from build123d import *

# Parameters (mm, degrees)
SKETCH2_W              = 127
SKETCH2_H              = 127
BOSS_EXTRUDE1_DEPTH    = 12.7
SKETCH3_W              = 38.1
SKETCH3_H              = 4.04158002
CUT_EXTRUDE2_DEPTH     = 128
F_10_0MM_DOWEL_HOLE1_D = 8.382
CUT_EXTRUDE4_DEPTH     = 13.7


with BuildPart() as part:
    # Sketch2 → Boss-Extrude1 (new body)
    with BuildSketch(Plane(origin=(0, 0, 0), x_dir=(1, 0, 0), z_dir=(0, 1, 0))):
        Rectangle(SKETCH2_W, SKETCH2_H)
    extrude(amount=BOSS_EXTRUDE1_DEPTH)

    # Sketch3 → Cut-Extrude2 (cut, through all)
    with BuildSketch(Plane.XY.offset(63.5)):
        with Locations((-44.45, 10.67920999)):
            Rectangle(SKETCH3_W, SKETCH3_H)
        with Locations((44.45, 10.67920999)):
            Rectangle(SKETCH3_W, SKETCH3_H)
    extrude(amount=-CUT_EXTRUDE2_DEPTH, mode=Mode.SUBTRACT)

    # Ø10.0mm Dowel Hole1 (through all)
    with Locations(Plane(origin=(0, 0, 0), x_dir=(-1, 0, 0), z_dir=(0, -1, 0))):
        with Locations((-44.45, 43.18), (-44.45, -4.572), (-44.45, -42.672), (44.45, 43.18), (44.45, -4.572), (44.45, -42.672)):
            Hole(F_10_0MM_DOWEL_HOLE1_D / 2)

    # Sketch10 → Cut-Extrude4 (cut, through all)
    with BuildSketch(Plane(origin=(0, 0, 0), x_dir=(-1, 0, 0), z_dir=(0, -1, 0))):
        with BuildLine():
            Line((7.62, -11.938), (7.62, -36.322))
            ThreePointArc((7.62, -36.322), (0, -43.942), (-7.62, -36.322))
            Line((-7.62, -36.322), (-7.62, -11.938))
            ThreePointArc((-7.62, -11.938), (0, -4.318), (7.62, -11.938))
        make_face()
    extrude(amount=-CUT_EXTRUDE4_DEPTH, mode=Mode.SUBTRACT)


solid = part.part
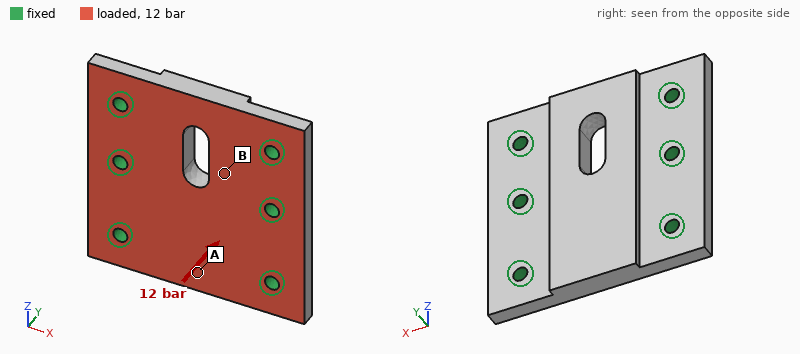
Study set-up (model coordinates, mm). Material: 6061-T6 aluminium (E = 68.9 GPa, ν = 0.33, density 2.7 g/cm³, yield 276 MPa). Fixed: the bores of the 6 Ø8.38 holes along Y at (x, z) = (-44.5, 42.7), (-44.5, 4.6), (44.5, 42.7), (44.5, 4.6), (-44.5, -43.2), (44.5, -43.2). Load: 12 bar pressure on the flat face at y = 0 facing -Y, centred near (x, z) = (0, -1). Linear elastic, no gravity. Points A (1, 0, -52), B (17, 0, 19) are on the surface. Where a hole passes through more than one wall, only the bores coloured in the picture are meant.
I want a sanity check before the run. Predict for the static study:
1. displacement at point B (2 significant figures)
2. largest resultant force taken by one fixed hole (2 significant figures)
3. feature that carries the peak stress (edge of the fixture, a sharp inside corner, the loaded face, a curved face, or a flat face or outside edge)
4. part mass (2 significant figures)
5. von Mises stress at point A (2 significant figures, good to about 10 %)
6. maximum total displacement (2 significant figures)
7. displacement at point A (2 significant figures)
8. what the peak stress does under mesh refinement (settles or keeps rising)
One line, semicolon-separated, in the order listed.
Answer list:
29 µm; 3.5 kN; edge of the fixture; 420 g; 18 MPa; 43 µm; 37 µm; keeps rising
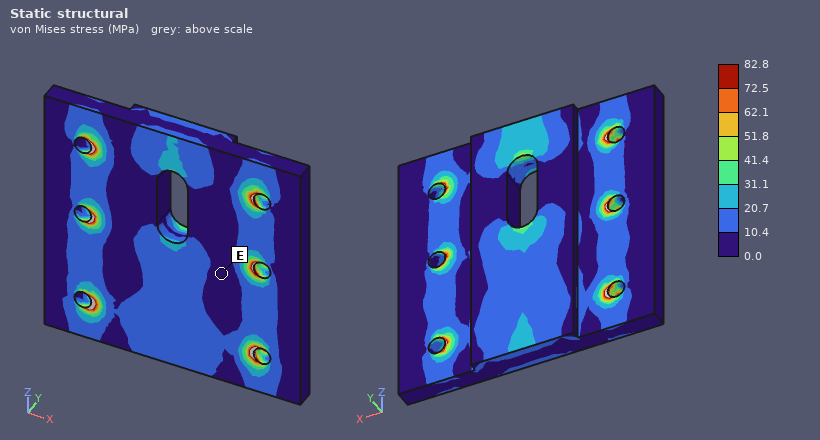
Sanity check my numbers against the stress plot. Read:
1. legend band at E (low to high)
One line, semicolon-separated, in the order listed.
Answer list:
0.0 to 10.4 MPa
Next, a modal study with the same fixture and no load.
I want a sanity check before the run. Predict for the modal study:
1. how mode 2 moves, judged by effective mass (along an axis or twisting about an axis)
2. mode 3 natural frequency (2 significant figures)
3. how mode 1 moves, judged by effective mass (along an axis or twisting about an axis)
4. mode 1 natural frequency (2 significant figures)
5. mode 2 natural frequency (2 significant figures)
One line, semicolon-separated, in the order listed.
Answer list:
twisting about X; 7800 Hz; along Y; 5500 Hz; 5900 Hz
